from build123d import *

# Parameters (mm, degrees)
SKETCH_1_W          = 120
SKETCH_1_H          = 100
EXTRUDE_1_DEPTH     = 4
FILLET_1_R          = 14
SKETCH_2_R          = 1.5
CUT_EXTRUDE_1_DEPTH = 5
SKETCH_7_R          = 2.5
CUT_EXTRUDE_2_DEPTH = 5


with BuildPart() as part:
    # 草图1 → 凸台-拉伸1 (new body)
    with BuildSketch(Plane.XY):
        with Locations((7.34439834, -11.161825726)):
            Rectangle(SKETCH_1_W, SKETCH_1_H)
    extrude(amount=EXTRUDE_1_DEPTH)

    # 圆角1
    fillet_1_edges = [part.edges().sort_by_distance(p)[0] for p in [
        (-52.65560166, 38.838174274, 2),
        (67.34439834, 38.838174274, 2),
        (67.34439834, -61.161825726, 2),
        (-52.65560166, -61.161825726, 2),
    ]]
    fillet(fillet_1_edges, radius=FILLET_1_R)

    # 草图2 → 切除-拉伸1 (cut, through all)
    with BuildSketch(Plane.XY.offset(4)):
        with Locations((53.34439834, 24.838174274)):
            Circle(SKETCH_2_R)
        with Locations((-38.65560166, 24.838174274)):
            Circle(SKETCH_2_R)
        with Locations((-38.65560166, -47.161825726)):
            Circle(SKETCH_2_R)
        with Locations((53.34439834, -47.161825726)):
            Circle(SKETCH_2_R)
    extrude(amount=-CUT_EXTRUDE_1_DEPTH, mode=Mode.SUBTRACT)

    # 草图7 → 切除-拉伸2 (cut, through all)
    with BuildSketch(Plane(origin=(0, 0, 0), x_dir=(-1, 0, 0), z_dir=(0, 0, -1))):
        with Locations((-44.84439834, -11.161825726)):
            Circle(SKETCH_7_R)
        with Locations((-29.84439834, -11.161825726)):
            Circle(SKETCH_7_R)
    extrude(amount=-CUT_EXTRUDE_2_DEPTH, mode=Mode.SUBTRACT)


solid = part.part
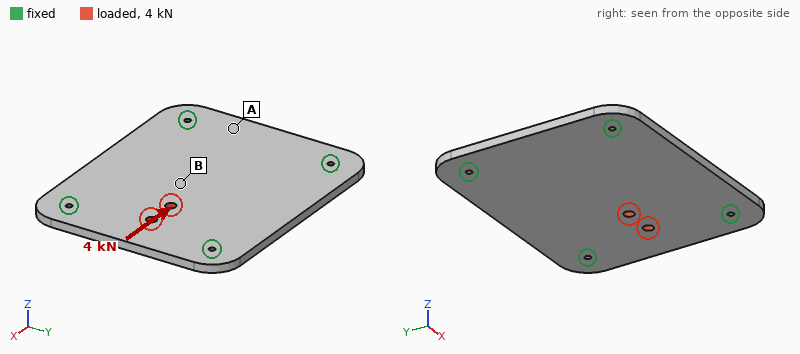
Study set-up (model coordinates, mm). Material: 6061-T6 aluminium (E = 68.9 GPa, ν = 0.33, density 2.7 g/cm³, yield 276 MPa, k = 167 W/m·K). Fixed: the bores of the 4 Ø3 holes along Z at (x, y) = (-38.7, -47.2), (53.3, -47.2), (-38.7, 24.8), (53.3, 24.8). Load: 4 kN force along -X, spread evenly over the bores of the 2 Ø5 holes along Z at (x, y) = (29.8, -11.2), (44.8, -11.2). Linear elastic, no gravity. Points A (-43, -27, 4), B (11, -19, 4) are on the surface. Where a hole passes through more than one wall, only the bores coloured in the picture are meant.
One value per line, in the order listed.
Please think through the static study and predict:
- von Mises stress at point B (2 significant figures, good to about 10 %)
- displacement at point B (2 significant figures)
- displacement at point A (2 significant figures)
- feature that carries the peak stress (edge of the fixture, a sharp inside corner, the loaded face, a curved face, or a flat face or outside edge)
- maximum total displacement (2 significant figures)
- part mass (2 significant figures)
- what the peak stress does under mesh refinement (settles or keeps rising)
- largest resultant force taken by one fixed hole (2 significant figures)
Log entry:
13 MPa
7.9 µm
3.5 µm
edge of the fixture
17 µm
130 g
keeps rising
1.2 kN
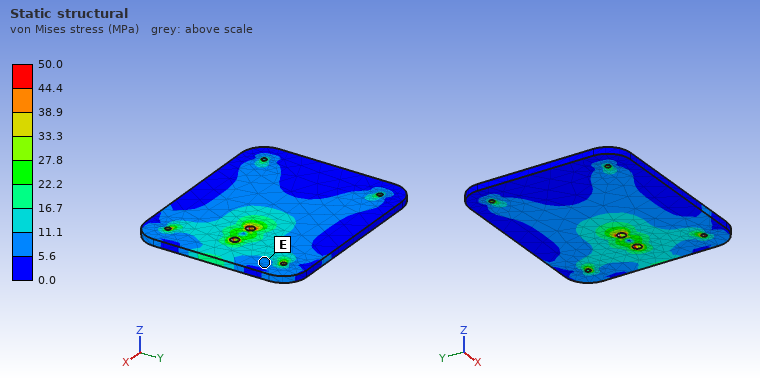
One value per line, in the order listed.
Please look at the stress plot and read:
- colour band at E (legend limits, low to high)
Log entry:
5.6 to 11.1 MPa
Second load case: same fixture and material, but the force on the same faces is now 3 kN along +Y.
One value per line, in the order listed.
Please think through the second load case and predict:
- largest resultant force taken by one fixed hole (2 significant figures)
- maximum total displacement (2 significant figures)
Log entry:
1.2 kN
9.4 µm
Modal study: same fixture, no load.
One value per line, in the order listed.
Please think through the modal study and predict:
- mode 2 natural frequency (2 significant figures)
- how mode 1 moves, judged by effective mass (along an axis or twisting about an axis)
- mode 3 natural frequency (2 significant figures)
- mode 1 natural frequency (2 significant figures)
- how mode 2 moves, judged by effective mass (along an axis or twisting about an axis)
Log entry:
2600 Hz
along Z
3200 Hz
1800 Hz
twisting about X
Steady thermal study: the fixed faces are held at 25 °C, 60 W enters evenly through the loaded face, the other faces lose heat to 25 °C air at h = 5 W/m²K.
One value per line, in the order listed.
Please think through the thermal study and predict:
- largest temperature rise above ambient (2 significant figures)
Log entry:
44 K
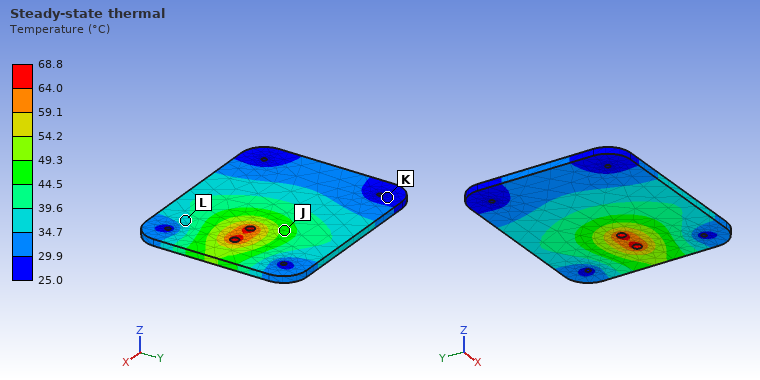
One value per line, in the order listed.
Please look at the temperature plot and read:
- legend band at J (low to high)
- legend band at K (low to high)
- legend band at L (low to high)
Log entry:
44.5 to 49.3 °C
25.0 to 29.9 °C
34.7 to 39.6 °C
